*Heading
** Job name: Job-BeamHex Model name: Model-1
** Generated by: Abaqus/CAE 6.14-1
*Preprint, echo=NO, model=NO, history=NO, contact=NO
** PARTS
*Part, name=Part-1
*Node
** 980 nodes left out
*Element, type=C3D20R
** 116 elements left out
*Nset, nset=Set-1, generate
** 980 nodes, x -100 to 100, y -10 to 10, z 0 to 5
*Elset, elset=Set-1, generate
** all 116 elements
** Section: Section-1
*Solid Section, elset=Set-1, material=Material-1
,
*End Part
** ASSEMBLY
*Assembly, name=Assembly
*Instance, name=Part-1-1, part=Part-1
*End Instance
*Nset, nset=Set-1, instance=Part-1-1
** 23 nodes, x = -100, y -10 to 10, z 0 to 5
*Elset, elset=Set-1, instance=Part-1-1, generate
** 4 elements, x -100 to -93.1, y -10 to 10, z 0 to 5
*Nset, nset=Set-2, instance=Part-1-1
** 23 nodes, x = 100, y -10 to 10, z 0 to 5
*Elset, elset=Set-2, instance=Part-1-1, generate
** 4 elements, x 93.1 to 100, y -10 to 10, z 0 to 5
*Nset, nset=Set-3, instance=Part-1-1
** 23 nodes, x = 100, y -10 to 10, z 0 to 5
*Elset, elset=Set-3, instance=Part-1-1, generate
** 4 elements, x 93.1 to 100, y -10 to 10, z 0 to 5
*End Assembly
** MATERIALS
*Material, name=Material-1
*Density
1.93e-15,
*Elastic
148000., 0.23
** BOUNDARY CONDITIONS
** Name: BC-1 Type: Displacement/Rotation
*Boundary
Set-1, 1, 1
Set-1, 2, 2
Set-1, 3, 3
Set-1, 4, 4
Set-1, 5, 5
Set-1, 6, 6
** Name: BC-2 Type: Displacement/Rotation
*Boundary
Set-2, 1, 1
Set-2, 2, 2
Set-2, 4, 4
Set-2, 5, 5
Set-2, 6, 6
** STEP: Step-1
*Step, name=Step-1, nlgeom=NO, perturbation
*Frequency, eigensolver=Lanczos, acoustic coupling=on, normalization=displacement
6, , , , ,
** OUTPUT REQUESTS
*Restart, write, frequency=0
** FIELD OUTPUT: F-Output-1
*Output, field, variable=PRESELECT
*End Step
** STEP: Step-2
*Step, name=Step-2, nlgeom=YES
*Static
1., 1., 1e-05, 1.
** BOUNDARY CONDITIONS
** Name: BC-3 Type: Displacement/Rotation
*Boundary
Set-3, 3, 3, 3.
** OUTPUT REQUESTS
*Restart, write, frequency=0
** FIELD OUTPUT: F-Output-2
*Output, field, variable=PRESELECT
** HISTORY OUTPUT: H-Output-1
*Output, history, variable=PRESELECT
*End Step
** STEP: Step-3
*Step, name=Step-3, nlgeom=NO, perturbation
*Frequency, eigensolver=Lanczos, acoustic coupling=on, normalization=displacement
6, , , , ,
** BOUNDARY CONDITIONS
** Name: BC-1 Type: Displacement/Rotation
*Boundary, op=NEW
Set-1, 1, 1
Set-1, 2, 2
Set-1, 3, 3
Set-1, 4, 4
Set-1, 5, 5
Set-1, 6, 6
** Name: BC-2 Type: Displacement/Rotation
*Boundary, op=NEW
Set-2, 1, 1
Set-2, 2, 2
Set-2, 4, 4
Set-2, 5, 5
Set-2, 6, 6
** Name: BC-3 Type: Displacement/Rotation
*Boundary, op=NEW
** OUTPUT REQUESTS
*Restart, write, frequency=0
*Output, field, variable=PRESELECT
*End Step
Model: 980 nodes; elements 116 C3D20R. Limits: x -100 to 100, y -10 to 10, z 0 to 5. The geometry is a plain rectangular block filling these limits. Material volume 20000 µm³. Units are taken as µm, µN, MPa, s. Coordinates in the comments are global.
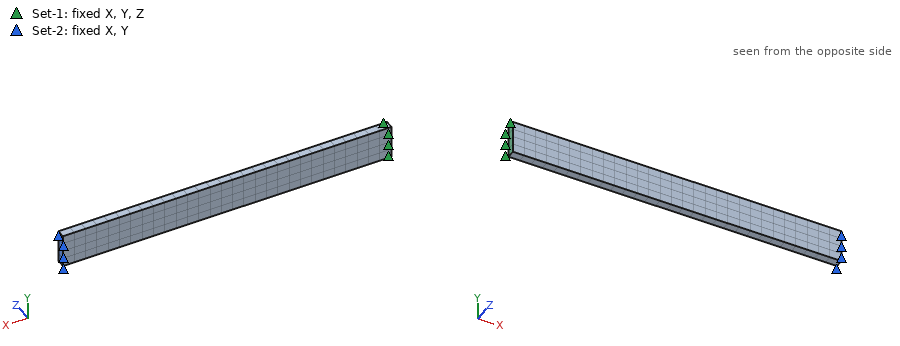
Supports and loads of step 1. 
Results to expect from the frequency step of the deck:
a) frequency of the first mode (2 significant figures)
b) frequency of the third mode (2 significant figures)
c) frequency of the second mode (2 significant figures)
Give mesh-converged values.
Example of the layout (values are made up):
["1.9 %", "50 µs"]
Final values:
["2.8e+05 Hz", "3.7e+06 Hz", "1.5e+06 Hz"]
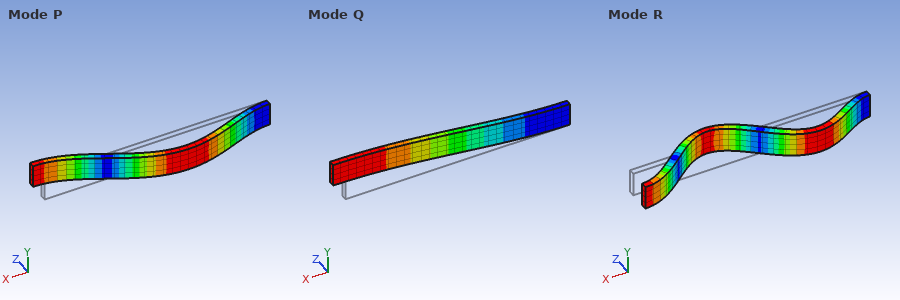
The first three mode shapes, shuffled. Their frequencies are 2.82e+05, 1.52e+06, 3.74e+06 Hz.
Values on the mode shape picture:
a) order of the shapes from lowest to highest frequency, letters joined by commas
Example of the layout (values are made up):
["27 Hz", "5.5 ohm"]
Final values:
["Q, P, R"]
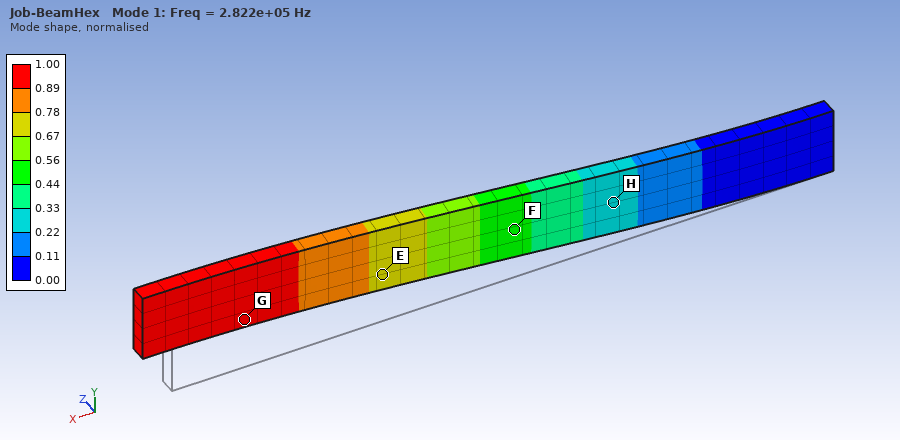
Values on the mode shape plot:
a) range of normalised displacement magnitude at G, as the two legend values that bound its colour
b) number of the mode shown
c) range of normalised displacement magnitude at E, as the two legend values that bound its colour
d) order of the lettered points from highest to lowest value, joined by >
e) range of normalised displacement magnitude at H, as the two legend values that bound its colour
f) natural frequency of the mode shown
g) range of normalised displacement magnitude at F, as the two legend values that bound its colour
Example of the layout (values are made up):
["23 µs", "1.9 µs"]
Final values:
["0.89 to 1.00", "1", "0.67 to 0.78", "G > E > F > H", "0.22 to 0.33", "2.822e+05 Hz", "0.44 to 0.56"]
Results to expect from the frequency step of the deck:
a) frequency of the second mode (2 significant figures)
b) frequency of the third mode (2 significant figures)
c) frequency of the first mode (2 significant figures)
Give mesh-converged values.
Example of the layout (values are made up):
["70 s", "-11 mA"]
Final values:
["1.6e+06 Hz", "3.8e+06 Hz", "3.7e+05 Hz"]
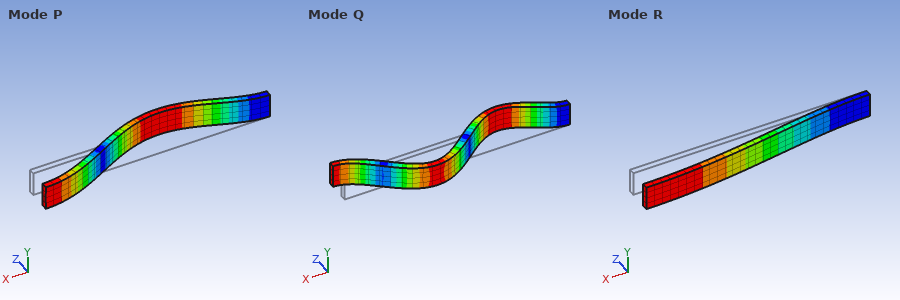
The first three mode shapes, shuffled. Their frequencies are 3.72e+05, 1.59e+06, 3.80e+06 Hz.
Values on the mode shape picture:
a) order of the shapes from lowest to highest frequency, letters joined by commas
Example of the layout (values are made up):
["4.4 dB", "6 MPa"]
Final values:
["R, P, Q"]
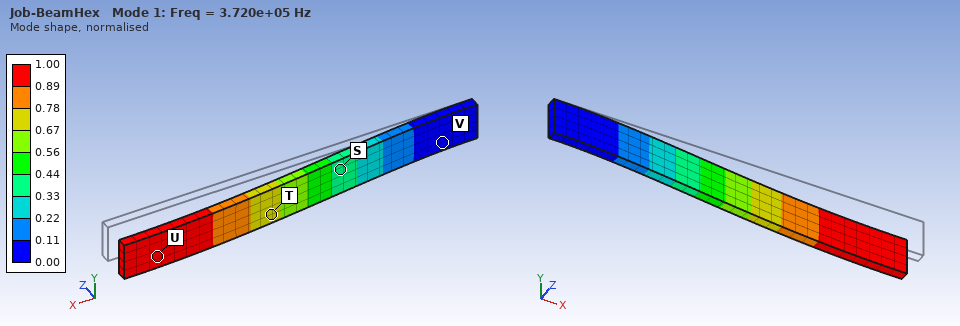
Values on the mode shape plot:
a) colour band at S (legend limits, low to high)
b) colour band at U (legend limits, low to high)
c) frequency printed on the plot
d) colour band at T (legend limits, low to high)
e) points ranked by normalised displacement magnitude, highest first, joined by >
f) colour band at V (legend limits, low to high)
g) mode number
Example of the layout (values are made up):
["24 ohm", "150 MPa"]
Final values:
["0.33 to 0.44", "0.89 to 1.00", "3.720e+05 Hz", "0.67 to 0.78", "U > T > S > V", "0.00 to 0.11", "1"]
